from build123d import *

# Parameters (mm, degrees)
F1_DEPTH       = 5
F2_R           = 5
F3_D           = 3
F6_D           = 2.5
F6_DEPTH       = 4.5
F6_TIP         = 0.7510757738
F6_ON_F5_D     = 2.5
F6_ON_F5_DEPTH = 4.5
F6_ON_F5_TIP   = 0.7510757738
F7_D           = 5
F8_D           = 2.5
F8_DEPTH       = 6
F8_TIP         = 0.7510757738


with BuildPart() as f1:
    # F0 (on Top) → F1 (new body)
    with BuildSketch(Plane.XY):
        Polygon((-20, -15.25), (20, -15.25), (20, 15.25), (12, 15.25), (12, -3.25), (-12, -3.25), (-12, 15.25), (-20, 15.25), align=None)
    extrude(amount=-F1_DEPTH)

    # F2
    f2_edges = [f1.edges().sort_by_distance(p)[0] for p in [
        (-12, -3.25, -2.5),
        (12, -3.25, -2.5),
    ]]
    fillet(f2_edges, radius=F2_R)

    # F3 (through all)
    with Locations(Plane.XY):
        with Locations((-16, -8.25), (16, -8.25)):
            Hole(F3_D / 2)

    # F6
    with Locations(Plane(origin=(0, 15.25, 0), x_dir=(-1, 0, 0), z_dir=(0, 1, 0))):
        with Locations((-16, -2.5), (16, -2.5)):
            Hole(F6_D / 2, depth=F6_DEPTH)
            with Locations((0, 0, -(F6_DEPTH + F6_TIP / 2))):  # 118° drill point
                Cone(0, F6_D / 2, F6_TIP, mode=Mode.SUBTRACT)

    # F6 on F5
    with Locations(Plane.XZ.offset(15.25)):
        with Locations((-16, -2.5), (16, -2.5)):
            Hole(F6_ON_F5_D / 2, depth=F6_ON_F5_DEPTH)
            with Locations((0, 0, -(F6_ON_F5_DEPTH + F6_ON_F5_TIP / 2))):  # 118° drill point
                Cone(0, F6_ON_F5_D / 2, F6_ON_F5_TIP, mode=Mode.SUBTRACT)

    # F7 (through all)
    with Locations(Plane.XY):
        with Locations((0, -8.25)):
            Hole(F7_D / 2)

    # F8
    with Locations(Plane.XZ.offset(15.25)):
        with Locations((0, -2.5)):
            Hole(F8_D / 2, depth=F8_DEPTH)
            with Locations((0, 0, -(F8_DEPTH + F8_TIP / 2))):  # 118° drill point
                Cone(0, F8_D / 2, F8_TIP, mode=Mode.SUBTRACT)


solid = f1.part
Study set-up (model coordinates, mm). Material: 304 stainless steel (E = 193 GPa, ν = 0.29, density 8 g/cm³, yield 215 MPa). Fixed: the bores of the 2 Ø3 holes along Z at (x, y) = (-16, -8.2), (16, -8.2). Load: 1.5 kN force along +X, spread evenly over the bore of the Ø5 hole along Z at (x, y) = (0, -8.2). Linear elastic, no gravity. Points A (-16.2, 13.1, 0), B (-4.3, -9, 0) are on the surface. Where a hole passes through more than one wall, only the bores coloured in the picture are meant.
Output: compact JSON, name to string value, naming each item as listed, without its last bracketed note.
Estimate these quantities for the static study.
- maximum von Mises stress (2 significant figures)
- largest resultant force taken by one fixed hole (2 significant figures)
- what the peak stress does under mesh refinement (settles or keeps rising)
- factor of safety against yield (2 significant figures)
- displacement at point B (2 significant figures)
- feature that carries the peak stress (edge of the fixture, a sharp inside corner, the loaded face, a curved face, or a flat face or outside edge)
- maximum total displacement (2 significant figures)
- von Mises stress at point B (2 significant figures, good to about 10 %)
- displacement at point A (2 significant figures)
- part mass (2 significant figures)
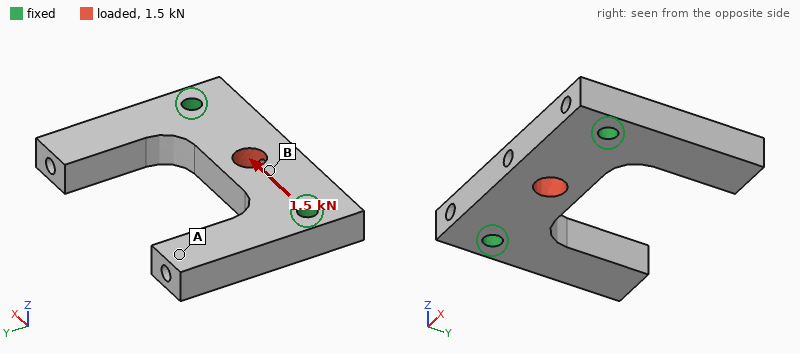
{"maximum von Mises stress": "46 MPa", "largest resultant force taken by one fixed hole": "750 N", "what the peak stress does under mesh refinement": "settles", "factor of safety against yield": "4.7", "displacement at point B": "1.0 µm", "feature that carries the peak stress": "the loaded face", "maximum total displacement": "1.4 µm", "von Mises stress at point B": "20 MPa", "displacement at point A": "0.92 µm", "part mass": "29 g"}
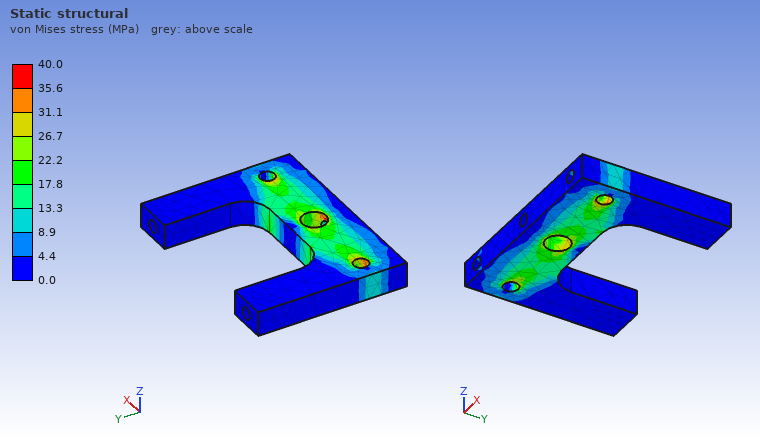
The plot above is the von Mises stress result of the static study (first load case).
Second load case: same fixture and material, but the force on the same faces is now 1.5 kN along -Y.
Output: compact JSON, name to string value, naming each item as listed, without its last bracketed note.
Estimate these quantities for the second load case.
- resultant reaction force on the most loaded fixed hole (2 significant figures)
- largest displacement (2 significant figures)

{"resultant reaction force on the most loaded fixed hole": "770 N", "largest displacement": "9.4 µm"}
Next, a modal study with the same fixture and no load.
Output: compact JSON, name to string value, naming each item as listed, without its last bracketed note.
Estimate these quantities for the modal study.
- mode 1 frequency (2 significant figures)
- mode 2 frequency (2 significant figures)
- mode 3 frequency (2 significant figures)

{"mode 1 frequency": "8000 Hz", "mode 2 frequency": "8100 Hz", "mode 3 frequency": "12 kHz"}
